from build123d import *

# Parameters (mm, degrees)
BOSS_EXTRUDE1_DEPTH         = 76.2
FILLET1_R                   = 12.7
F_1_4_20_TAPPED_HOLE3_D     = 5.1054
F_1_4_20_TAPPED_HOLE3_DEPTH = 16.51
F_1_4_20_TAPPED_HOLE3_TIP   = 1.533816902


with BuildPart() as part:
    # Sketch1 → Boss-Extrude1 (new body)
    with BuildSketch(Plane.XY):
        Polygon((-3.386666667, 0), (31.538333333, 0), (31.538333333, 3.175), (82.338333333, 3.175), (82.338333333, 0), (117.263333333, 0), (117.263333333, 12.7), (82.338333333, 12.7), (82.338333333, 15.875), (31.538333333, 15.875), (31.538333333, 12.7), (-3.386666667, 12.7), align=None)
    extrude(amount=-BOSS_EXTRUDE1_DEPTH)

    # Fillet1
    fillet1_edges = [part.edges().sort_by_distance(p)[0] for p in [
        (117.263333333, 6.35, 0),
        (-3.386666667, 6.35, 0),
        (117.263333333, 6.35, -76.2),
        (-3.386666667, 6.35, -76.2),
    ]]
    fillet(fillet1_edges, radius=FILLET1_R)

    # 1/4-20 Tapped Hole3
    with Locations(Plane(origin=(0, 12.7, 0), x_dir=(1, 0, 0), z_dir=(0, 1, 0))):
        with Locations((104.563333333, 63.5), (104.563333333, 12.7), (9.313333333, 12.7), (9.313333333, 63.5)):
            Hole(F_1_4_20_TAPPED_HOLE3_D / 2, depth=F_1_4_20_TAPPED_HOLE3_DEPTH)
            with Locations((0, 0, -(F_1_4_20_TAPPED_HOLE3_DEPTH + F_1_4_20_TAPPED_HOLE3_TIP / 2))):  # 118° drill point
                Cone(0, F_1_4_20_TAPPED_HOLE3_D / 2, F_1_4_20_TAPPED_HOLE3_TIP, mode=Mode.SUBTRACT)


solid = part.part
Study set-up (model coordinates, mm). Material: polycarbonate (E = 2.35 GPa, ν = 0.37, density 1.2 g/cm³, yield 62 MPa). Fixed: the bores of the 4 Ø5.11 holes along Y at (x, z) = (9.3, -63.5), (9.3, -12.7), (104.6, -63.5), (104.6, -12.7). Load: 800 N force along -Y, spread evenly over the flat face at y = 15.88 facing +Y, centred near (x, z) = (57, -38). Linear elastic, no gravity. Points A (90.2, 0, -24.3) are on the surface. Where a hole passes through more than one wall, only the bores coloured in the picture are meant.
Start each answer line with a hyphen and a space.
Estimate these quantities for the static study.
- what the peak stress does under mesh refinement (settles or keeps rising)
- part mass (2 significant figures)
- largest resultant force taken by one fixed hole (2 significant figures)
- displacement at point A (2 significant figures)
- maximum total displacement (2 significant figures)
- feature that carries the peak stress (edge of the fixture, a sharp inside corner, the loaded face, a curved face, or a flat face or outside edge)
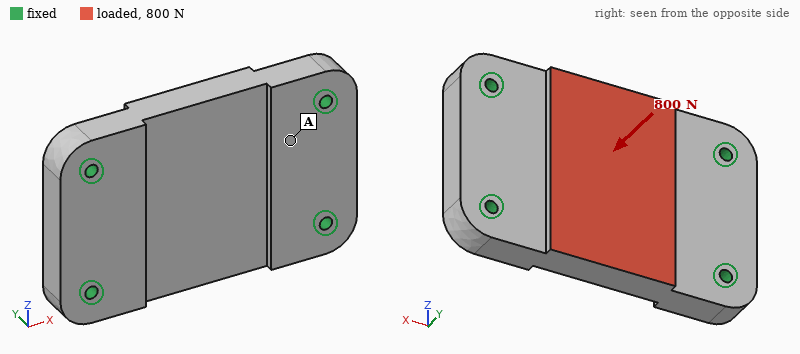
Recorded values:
- keeps rising
- 140 g
- 280 N
- 0.056 mm
- 0.14 mm
- edge of the fixture
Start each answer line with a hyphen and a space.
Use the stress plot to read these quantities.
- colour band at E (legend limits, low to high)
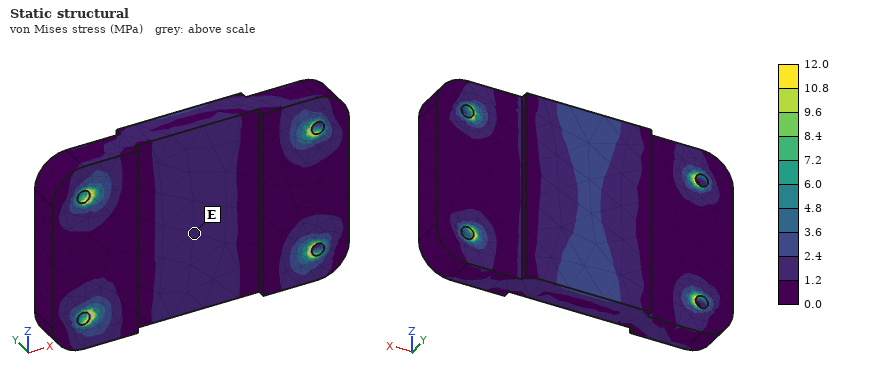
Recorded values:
- 1.2 to 2.4 MPa
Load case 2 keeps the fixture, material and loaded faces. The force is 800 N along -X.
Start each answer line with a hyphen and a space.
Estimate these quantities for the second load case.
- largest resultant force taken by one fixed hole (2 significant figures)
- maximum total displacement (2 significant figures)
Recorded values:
- 210 N
- 13 µm
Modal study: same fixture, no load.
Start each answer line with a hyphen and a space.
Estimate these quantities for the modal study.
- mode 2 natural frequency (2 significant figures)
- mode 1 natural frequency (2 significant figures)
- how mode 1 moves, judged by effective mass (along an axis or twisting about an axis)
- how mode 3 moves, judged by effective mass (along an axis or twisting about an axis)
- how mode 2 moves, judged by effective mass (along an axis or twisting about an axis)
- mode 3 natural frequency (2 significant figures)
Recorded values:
- 2100 Hz
- 1600 Hz
- along Y
- along Z
- twisting about X
- 3500 Hz
